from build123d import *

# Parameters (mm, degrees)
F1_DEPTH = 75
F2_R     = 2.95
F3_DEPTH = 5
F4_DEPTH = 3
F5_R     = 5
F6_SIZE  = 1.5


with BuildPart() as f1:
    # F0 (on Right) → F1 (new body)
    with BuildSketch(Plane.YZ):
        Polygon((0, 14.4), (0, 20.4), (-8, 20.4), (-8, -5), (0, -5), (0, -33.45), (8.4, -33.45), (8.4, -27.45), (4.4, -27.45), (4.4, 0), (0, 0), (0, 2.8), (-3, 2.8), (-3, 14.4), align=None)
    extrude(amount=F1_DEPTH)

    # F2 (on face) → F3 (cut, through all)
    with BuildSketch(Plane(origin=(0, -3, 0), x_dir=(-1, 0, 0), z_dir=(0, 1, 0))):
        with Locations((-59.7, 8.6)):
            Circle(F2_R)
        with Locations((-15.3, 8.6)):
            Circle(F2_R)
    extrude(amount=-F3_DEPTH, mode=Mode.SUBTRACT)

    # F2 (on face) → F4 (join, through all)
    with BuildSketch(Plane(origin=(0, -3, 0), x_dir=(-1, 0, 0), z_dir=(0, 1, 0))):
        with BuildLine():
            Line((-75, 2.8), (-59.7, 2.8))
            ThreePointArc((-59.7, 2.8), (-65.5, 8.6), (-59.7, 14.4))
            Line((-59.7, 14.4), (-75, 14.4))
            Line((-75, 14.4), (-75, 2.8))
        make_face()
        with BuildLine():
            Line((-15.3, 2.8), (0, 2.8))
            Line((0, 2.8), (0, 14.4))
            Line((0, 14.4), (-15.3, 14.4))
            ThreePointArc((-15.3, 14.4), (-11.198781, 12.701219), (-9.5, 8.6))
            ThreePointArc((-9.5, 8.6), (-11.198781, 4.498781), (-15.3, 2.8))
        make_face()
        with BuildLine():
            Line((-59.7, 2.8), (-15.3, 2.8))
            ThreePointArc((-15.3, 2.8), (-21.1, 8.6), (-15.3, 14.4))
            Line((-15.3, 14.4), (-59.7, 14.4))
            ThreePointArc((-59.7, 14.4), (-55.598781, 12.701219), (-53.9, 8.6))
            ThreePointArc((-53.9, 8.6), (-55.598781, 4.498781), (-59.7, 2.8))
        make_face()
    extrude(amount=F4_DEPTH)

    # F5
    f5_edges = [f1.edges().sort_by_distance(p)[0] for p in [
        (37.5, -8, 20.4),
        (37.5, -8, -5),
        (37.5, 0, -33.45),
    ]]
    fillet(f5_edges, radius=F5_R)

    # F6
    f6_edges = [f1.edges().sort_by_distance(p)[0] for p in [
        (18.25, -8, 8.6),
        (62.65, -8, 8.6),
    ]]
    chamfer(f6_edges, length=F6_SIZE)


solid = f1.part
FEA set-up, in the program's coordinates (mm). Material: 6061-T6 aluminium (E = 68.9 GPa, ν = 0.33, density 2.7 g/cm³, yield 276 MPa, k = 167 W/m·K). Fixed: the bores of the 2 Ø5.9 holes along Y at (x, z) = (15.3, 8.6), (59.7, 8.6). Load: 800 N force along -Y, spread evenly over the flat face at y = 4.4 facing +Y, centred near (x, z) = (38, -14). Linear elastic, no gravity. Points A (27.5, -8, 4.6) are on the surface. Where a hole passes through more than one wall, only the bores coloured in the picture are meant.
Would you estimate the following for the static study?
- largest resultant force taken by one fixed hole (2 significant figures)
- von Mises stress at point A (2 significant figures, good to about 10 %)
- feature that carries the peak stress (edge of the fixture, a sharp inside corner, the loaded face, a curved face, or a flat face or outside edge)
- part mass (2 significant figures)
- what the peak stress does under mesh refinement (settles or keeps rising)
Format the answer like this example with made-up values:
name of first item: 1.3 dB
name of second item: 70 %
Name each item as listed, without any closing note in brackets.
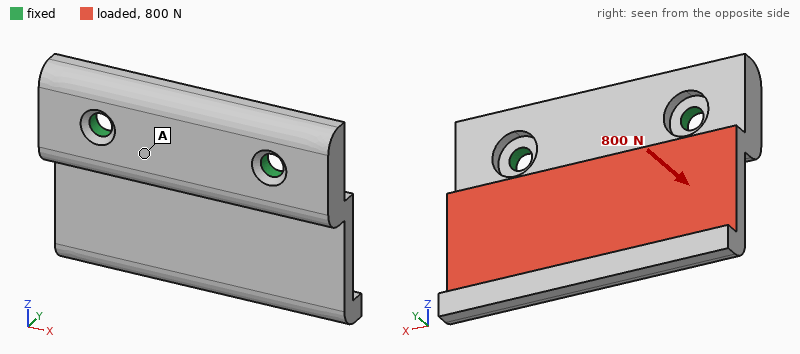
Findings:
largest resultant force taken by one fixed hole: 410 N
von Mises stress at point A: 15 MPa
feature that carries the peak stress: edge of the fixture
part mass: 70 g
what the peak stress does under mesh refinement: keeps rising
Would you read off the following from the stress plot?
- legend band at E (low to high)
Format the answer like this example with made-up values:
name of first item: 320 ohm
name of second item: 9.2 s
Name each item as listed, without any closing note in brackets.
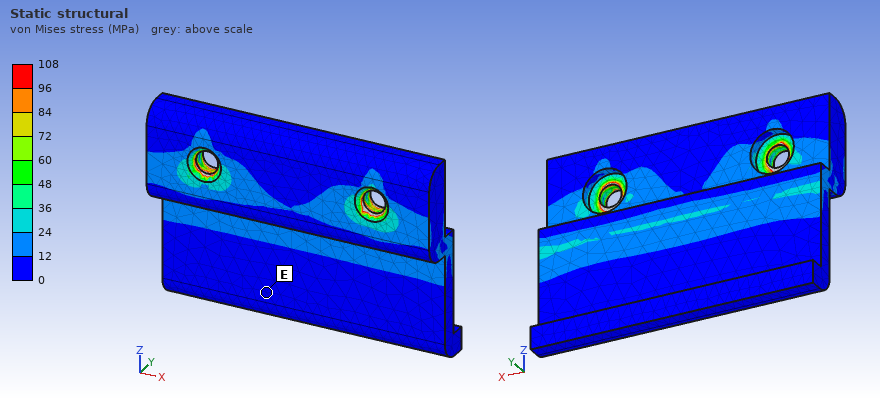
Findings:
legend band at E: 0 to 12 MPa
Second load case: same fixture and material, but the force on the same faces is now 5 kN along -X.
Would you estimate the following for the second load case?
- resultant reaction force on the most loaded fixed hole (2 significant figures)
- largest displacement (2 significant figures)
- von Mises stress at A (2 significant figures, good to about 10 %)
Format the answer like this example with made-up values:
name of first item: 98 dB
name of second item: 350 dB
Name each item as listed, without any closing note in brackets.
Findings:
resultant reaction force on the most loaded fixed hole: 3.5 kN
largest displacement: 45 µm
von Mises stress at A: 20 MPa
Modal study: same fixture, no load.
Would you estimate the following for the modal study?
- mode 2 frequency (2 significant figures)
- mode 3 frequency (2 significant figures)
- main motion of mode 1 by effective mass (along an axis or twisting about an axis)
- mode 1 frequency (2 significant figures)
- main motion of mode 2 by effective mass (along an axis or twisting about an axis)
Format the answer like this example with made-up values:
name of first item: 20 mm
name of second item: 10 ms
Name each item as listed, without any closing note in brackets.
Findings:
mode 2 frequency: 3500 Hz
mode 3 frequency: 8200 Hz
main motion of mode 1 by effective mass: along Y
mode 1 frequency: 2000 Hz
main motion of mode 2 by effective mass: twisting about Z
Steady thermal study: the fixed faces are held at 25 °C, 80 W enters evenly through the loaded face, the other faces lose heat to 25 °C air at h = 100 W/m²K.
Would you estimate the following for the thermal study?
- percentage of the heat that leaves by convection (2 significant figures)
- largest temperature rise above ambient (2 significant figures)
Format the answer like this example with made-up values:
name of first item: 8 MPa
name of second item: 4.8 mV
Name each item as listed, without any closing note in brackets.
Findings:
percentage of the heat that leaves by convection: 18 %
largest temperature rise above ambient: 30 K
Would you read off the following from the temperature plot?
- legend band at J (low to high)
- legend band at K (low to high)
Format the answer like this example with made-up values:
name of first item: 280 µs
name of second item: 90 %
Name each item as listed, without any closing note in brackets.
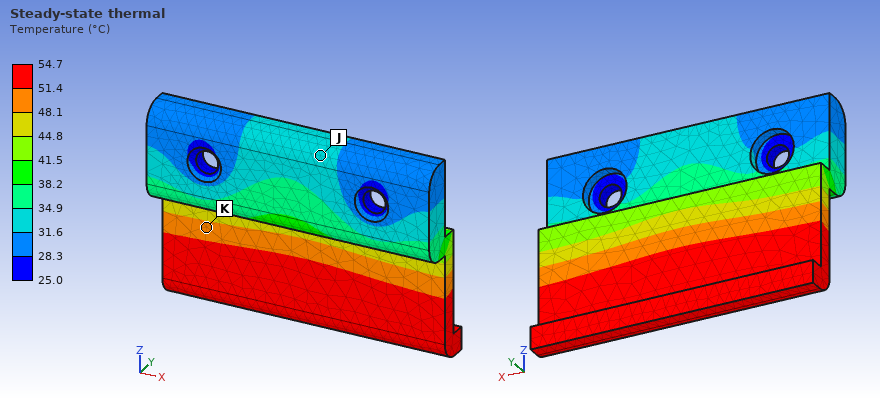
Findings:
legend band at J: 31.6 to 34.9 °C
legend band at K: 48.1 to 51.4 °C
